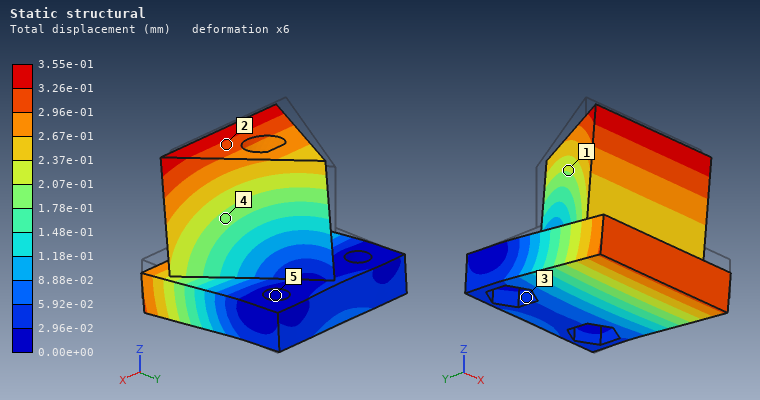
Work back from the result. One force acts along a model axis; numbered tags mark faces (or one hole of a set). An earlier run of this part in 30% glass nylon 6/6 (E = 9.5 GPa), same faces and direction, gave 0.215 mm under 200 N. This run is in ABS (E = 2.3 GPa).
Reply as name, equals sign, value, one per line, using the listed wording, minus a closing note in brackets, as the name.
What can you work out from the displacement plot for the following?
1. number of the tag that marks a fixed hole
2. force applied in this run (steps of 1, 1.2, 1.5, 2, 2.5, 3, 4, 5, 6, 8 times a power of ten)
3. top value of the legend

number of the tag that marks a fixed hole = 5
force applied in this run = 80 N
top value of the legend = 3.55e-01 mm
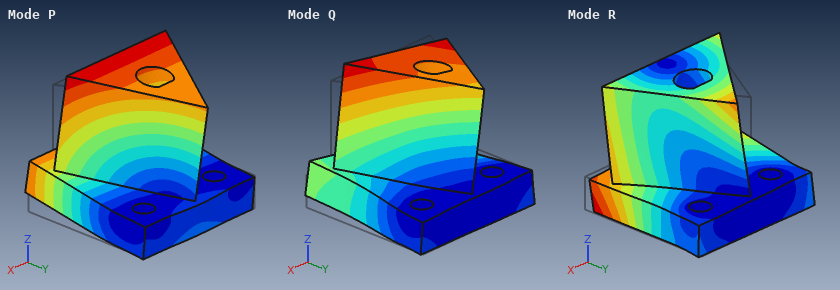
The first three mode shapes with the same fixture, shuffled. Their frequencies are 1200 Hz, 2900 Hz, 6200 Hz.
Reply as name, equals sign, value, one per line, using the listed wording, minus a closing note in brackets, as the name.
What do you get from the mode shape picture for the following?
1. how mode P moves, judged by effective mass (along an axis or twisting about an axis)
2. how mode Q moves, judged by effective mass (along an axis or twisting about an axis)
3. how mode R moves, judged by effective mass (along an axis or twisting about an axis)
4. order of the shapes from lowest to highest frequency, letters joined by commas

how mode P moves, judged by effective mass = along Z
how mode Q moves, judged by effective mass = along X
how mode R moves, judged by effective mass = along X
order of the shapes from lowest to highest frequency, letters joined by commas = P, Q, R
